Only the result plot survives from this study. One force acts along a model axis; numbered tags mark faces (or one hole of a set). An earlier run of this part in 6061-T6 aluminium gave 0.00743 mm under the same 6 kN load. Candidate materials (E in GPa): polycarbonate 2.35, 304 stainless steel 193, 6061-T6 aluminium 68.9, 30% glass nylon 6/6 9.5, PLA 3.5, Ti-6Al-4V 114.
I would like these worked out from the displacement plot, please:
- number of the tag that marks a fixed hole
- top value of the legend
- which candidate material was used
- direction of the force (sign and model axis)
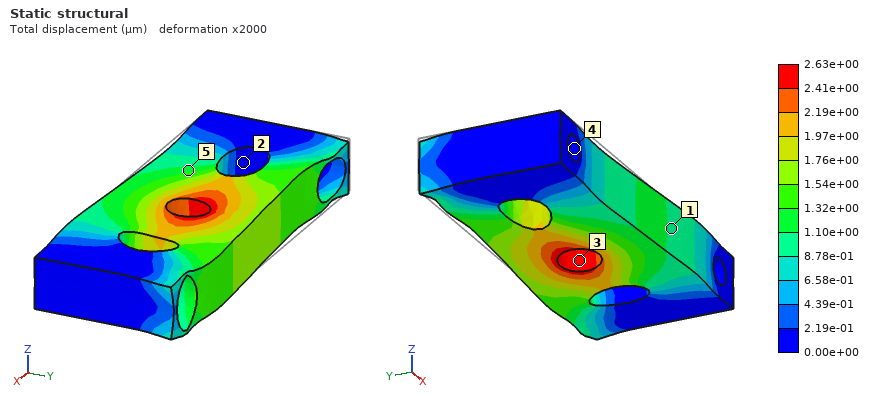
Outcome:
4
2.63e+00 µm
304 stainless steel
+X
